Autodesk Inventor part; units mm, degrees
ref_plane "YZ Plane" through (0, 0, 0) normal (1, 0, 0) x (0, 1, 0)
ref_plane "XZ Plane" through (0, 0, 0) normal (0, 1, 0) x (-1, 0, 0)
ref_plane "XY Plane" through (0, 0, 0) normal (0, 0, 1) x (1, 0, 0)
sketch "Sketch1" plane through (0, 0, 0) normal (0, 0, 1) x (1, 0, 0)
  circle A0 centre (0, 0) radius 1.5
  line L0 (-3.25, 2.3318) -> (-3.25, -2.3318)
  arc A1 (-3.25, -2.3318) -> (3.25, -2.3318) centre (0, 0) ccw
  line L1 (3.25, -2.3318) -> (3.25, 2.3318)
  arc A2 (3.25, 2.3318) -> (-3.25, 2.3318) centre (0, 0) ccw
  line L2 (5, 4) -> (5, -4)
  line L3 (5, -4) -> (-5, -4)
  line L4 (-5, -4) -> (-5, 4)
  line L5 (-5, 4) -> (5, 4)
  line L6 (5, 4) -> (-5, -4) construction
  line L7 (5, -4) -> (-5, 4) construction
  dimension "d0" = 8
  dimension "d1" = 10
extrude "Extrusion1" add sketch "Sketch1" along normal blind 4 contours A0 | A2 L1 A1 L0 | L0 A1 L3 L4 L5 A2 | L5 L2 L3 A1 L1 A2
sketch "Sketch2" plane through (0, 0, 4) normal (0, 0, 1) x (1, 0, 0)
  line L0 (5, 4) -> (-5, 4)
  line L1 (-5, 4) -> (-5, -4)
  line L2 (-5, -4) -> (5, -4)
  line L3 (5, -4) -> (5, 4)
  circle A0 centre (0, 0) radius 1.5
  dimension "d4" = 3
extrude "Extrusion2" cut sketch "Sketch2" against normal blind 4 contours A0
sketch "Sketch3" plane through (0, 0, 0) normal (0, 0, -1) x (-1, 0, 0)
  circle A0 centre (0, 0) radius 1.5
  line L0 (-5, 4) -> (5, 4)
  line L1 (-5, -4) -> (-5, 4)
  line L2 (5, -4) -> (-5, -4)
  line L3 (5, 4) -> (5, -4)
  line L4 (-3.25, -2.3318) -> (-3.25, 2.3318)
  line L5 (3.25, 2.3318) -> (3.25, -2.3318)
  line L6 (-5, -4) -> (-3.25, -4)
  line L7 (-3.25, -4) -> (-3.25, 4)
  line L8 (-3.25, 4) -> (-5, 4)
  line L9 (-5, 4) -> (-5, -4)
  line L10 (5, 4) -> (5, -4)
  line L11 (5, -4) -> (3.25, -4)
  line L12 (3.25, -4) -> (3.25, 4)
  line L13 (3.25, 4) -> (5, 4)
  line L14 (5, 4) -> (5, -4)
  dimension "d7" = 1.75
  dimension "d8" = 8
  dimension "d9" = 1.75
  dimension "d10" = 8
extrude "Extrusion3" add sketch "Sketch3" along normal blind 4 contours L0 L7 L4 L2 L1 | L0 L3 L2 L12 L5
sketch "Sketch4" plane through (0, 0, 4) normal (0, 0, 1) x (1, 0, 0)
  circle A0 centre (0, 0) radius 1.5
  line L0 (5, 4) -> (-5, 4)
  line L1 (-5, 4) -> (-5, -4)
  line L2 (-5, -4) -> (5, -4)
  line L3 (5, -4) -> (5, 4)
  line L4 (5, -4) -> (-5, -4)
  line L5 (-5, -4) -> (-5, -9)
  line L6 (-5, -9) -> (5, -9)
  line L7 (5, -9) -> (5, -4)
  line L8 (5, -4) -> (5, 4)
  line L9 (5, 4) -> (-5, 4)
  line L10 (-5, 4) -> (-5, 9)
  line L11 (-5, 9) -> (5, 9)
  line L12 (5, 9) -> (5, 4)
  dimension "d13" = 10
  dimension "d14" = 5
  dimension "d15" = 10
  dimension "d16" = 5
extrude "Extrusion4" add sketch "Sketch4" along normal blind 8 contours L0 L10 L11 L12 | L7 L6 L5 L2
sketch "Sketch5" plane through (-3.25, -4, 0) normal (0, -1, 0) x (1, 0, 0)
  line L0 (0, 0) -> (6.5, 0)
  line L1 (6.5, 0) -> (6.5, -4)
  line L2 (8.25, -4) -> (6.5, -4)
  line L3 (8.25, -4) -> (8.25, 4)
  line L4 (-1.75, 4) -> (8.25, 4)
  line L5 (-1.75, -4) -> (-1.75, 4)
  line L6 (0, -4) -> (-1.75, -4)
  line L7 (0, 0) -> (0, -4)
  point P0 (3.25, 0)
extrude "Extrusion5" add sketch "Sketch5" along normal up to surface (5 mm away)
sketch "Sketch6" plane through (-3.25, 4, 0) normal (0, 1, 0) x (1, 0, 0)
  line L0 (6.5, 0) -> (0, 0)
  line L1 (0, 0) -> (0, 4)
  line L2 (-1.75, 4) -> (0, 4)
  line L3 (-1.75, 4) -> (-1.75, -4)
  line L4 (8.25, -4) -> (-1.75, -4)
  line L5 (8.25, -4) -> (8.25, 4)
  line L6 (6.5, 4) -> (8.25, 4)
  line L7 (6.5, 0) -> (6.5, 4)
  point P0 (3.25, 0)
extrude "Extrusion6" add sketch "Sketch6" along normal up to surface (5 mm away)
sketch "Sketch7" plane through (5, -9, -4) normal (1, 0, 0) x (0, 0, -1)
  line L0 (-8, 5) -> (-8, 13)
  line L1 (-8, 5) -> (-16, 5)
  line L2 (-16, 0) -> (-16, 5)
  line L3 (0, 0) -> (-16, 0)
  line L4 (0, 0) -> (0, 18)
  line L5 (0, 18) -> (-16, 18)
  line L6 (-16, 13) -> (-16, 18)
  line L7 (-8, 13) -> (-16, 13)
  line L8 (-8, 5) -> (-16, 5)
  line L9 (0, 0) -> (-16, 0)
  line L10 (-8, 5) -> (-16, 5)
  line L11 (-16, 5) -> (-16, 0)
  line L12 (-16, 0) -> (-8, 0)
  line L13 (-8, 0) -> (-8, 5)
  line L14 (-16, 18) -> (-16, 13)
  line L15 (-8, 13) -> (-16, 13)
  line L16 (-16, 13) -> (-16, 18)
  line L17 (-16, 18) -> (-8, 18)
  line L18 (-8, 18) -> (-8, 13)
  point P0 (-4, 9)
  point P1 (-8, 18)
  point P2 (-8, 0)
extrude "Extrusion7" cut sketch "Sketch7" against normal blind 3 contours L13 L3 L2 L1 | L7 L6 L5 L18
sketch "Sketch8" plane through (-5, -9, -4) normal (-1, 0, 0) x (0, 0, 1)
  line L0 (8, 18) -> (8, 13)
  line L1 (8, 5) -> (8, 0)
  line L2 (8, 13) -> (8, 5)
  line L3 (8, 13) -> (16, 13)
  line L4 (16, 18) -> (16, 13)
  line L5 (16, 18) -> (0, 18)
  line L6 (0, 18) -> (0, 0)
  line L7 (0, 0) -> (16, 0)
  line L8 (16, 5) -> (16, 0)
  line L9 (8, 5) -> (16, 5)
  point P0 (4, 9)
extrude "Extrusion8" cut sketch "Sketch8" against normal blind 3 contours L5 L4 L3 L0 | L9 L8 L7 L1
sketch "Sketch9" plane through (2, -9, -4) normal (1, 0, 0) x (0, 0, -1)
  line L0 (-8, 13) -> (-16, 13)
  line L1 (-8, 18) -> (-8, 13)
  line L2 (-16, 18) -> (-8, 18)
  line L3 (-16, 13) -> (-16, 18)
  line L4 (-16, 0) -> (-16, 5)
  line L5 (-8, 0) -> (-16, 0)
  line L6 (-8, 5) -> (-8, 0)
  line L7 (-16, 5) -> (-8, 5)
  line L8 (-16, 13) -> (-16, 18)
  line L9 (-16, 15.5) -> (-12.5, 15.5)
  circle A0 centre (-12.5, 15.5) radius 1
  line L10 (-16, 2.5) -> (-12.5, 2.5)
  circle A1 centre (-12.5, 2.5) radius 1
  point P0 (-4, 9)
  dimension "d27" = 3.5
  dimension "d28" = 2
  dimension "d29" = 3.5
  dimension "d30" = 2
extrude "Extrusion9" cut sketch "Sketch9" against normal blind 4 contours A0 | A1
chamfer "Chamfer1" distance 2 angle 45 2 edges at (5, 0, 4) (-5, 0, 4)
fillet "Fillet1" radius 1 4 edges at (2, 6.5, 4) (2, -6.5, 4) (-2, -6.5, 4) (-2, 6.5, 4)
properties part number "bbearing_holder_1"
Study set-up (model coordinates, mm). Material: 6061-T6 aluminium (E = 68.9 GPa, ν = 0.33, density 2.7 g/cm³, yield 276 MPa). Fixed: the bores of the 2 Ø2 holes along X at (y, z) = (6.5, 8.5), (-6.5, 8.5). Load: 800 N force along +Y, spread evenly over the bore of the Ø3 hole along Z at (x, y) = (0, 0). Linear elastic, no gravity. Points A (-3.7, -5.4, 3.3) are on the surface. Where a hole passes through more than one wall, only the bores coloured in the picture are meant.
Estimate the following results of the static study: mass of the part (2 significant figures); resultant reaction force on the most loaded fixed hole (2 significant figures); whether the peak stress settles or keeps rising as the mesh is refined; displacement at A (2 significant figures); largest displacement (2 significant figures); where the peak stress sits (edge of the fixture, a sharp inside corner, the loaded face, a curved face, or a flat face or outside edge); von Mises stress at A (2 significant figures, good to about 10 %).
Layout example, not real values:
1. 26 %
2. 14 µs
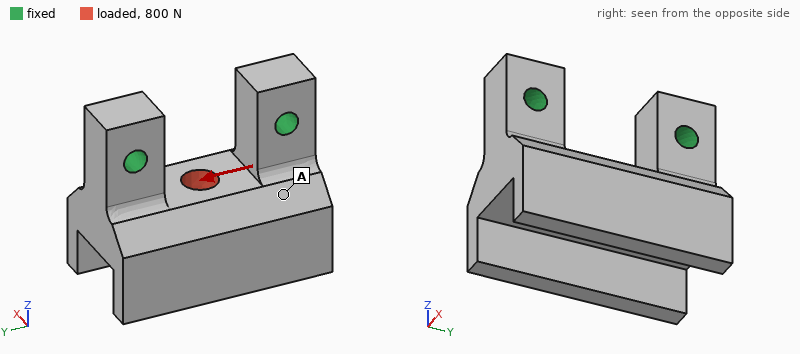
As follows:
1. 3.2 g
2. 460 N
3. keeps rising
4. 8.3 µm
5. 10 µm
6. edge of the fixture
7. 13 MPa
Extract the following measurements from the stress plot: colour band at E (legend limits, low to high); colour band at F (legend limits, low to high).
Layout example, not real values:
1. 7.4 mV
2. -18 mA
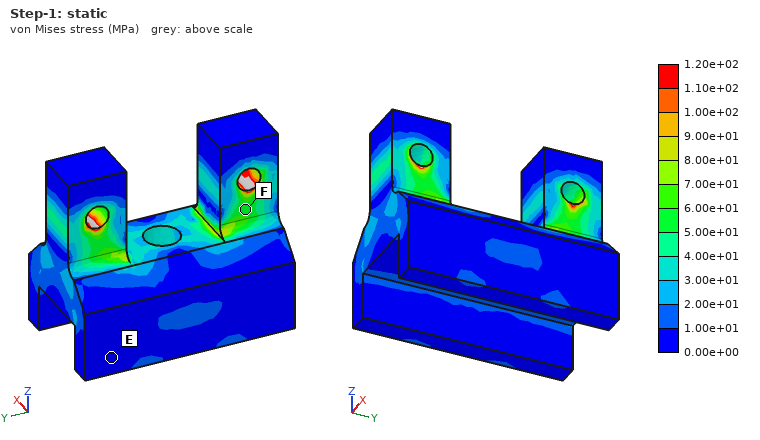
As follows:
1. 0.00e+00 to 1.00e+01 MPa
2. 5.00e+01 to 6.00e+01 MPa
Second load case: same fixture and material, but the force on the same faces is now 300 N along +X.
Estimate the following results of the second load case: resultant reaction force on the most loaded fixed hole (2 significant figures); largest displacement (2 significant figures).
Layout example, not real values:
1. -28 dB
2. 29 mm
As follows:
1. 150 N
2. 20 µm
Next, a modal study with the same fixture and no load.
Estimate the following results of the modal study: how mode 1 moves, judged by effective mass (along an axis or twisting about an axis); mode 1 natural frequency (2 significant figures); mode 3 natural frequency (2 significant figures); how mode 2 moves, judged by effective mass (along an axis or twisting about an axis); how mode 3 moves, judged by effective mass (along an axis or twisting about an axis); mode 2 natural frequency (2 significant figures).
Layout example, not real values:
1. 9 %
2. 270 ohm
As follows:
1. along X
2. 13 kHz
3. 29 kHz
4. twisting about Z
5. along Y
6. 27 kHz
